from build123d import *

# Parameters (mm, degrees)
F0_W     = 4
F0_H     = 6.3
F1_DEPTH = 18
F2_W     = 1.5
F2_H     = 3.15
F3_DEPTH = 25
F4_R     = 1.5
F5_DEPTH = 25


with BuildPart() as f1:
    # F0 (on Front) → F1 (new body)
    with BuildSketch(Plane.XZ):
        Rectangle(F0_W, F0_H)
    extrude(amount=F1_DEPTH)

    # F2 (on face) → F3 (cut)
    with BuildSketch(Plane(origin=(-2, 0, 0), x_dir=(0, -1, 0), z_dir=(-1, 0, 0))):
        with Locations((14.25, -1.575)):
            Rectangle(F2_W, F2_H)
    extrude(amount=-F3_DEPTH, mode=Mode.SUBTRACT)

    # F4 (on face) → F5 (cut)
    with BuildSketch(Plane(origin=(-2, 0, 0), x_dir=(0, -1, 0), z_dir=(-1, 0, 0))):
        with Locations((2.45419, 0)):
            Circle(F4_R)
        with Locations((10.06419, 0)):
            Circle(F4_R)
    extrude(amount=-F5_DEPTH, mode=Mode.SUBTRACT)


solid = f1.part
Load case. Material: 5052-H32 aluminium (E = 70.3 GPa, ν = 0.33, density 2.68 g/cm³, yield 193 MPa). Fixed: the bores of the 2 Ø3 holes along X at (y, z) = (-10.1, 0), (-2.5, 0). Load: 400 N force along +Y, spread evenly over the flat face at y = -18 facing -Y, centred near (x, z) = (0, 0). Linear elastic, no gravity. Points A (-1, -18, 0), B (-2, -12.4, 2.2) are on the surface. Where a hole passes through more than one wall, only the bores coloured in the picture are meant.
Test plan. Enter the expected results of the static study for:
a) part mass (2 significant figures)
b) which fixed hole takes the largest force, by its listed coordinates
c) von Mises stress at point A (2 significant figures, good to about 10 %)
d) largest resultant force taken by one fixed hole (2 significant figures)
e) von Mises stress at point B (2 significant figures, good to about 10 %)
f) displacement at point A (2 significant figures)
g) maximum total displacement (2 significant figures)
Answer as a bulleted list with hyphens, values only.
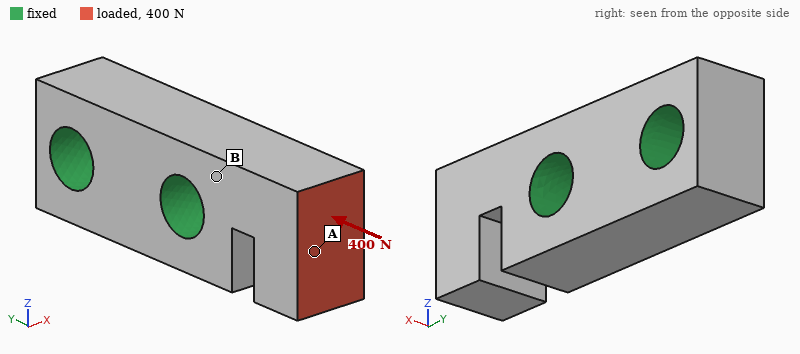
- 1.0 g
- (-10.1, 0)
- 52 MPa
- 390 N
- 26 MPa
- 15 µm
- 24 µm
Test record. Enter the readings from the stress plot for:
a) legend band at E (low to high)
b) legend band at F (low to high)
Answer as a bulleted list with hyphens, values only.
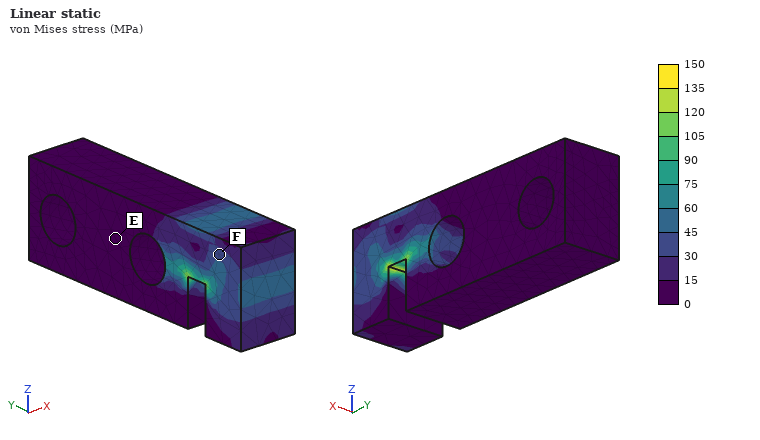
- 0 to 15 MPa
- 30 to 45 MPa
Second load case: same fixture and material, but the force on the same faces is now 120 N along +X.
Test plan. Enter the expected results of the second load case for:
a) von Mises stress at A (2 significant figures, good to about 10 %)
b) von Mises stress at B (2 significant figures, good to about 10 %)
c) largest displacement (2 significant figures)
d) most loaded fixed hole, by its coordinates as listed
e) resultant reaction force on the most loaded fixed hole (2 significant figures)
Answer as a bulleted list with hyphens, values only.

- 16 MPa
- 59 MPa
- 19 µm
- (-10.1, 0)
- 130 N
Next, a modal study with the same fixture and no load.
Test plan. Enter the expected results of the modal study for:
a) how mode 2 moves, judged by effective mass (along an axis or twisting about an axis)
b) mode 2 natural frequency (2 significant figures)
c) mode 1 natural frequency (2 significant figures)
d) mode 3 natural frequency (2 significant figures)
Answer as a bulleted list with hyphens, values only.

- along X
- 39 kHz
- 37 kHz
- 68 kHz
